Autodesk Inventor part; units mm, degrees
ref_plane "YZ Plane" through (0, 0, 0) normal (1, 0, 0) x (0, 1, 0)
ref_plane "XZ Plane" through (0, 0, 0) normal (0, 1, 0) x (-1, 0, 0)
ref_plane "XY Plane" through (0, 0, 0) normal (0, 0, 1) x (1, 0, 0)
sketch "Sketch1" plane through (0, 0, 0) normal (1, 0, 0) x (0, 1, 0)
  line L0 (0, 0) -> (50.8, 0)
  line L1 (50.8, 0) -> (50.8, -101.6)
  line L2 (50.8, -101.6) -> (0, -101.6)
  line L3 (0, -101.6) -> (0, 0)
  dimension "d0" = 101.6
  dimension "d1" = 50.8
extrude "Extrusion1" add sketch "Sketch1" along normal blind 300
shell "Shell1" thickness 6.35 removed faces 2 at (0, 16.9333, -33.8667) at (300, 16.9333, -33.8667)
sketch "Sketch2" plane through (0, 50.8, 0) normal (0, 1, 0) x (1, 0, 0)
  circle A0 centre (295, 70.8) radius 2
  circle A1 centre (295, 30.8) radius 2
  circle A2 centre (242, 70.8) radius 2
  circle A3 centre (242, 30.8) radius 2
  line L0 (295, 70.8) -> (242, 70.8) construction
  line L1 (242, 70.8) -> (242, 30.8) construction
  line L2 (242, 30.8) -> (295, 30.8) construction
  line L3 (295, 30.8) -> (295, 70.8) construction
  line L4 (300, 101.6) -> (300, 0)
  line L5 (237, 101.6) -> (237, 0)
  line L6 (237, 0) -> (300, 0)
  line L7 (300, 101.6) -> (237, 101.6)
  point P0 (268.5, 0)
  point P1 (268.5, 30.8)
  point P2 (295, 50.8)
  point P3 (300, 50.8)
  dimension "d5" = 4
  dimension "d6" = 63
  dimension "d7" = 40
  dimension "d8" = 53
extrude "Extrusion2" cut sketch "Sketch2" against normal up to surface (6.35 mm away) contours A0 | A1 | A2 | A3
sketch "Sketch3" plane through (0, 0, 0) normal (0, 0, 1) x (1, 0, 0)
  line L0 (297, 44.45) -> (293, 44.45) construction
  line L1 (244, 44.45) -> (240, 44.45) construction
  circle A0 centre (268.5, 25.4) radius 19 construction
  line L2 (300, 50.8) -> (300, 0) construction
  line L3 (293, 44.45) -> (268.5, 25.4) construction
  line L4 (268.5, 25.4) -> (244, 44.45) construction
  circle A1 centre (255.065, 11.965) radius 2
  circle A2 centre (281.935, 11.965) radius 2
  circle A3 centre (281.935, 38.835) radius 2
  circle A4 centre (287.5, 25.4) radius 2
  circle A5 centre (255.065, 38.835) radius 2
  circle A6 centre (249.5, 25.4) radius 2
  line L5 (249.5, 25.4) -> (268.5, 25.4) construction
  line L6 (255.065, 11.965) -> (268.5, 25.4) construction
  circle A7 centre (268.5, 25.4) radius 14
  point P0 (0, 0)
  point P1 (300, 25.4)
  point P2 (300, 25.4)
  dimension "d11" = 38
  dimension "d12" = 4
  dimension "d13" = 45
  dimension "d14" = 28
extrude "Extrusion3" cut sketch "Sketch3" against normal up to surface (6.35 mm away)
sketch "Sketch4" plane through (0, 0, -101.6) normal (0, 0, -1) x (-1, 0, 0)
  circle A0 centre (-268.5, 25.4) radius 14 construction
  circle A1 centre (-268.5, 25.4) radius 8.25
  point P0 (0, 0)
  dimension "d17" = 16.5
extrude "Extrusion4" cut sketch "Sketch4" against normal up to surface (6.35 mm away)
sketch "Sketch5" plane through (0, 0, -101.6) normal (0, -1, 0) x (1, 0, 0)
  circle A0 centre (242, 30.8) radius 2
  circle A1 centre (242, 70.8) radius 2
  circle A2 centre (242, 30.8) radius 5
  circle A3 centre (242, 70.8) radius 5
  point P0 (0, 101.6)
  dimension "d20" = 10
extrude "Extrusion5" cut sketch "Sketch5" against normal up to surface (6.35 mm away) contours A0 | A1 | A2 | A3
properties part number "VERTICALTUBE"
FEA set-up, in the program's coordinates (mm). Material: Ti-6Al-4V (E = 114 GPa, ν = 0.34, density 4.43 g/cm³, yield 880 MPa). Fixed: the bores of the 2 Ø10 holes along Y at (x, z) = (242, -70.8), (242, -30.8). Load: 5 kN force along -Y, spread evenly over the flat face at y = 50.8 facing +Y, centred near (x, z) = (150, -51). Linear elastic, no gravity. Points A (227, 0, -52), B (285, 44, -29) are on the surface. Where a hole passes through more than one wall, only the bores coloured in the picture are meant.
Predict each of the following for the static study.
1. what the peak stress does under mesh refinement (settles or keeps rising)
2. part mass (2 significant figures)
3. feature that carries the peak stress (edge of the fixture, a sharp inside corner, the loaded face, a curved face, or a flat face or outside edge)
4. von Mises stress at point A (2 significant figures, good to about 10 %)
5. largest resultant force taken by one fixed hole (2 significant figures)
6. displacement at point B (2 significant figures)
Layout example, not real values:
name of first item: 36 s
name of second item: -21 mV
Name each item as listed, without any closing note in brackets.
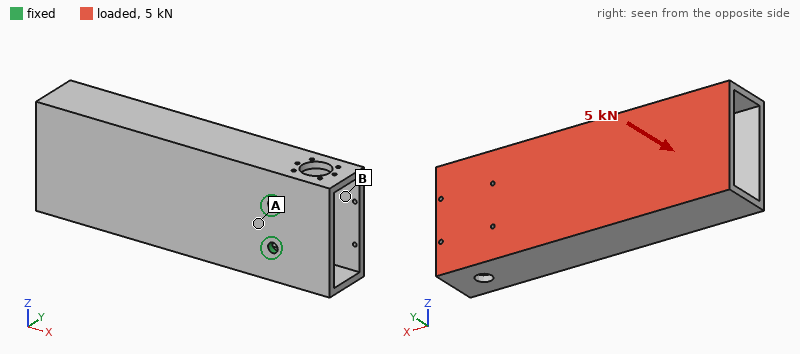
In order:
what the peak stress does under mesh refinement: keeps rising
part mass: 2.3 kg
feature that carries the peak stress: edge of the fixture
von Mises stress at point A: 200 MPa
largest resultant force taken by one fixed hole: 2.5 kN
displacement at point B: 0.83 mm
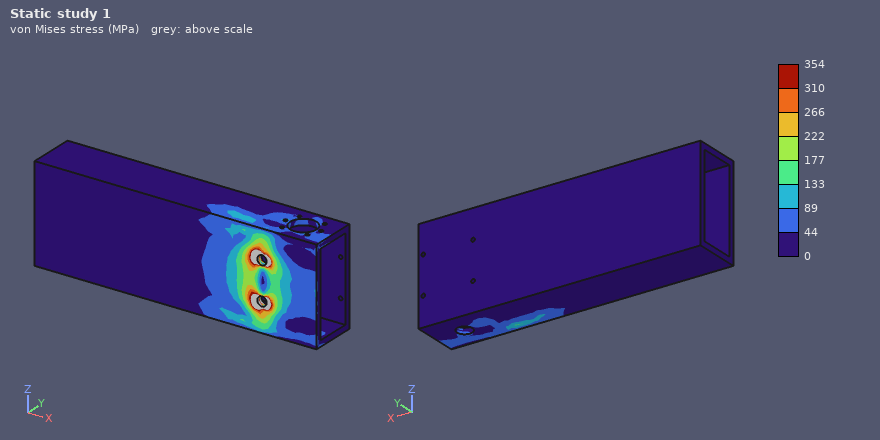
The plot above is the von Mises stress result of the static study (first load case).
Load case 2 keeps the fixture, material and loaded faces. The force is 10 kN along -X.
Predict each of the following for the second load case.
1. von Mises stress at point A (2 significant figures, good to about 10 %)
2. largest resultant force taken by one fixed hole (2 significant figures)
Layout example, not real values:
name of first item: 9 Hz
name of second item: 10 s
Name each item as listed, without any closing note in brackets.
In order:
von Mises stress at point A: 190 MPa
largest resultant force taken by one fixed hole: 5.0 kN
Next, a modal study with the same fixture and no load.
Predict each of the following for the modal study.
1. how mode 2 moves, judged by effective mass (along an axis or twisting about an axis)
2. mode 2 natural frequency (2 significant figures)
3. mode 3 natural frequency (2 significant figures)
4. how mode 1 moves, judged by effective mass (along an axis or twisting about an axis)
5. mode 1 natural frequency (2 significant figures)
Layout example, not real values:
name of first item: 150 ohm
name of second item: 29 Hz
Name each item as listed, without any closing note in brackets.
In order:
how mode 2 moves, judged by effective mass: along Z
mode 2 natural frequency: 540 Hz
mode 3 natural frequency: 750 Hz
how mode 1 moves, judged by effective mass: along Y
mode 1 natural frequency: 140 Hz
